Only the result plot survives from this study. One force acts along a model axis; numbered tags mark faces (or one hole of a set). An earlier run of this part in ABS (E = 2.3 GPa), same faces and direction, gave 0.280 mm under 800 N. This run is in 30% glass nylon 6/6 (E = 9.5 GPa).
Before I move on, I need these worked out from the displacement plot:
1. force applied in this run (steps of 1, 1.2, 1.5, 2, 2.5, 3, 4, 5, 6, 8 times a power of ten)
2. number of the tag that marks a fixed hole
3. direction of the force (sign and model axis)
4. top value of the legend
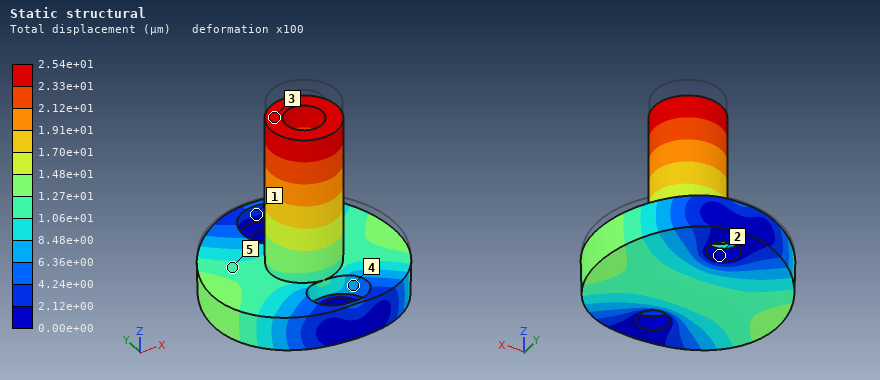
300 N
2
-Z
2.54e+01 µm
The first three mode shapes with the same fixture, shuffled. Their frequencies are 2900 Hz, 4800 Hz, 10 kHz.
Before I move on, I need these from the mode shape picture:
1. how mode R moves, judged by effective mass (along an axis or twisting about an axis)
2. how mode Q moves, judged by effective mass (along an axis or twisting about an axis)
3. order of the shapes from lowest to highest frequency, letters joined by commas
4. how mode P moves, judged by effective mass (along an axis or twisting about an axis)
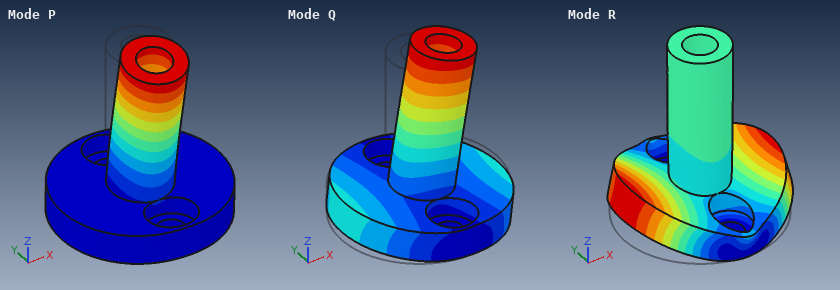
along Z
along X
Q, P, R
along Y
